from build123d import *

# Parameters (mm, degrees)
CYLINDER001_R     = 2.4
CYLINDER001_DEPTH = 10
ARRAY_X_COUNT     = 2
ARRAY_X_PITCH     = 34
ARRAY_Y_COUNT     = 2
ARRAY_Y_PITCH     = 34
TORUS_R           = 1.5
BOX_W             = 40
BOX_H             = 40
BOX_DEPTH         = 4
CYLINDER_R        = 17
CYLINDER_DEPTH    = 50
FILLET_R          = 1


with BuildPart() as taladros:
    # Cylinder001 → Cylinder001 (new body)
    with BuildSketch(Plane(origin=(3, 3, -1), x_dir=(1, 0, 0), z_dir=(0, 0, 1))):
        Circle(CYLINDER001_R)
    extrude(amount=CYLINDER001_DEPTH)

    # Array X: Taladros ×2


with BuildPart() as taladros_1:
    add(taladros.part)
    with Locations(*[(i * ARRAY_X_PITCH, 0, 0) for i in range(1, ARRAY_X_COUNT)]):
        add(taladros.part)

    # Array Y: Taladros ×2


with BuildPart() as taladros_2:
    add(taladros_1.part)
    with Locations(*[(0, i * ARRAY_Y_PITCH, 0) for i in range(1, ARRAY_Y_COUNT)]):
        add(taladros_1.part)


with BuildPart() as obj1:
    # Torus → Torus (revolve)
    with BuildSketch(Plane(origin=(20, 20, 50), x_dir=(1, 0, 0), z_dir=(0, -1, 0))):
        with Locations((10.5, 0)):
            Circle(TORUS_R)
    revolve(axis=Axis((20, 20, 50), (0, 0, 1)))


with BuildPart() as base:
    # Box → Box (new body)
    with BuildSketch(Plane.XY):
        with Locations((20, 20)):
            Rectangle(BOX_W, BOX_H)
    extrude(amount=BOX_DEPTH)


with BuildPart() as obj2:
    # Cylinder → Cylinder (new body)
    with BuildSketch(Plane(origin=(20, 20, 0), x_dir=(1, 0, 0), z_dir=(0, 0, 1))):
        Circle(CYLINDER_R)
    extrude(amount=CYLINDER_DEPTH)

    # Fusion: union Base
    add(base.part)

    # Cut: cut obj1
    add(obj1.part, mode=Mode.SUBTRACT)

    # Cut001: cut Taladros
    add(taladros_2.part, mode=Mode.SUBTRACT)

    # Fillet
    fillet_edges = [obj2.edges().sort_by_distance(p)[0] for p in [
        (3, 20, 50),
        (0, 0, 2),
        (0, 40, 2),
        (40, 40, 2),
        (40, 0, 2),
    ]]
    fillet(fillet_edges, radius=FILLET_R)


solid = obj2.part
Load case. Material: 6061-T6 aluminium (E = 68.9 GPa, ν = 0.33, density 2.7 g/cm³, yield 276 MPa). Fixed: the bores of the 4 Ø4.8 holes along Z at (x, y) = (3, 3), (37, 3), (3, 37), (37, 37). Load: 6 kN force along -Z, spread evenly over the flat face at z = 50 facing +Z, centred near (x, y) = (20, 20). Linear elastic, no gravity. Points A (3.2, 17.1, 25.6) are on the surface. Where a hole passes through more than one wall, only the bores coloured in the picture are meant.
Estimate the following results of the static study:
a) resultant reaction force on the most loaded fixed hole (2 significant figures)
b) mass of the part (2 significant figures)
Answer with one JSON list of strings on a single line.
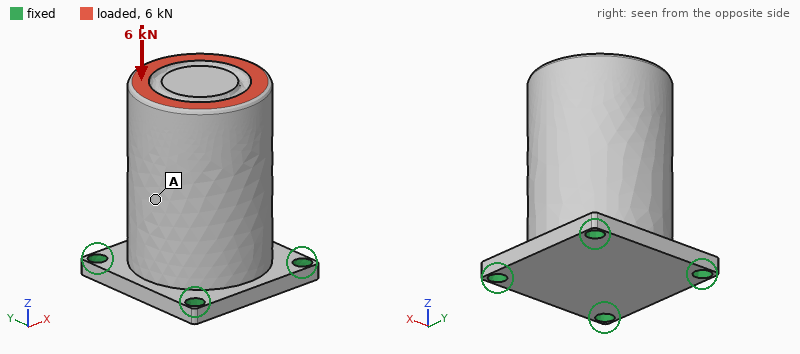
["1.6 kN", "130 g"]
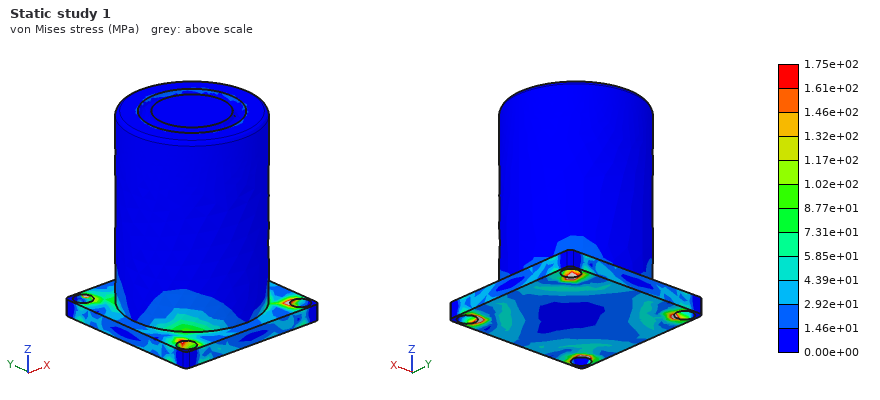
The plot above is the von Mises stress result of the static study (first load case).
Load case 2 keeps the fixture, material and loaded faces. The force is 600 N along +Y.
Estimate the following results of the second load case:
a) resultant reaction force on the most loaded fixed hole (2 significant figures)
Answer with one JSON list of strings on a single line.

["540 N"]
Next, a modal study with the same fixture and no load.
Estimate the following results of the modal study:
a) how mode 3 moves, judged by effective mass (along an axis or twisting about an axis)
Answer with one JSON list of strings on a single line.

["along Z"]
